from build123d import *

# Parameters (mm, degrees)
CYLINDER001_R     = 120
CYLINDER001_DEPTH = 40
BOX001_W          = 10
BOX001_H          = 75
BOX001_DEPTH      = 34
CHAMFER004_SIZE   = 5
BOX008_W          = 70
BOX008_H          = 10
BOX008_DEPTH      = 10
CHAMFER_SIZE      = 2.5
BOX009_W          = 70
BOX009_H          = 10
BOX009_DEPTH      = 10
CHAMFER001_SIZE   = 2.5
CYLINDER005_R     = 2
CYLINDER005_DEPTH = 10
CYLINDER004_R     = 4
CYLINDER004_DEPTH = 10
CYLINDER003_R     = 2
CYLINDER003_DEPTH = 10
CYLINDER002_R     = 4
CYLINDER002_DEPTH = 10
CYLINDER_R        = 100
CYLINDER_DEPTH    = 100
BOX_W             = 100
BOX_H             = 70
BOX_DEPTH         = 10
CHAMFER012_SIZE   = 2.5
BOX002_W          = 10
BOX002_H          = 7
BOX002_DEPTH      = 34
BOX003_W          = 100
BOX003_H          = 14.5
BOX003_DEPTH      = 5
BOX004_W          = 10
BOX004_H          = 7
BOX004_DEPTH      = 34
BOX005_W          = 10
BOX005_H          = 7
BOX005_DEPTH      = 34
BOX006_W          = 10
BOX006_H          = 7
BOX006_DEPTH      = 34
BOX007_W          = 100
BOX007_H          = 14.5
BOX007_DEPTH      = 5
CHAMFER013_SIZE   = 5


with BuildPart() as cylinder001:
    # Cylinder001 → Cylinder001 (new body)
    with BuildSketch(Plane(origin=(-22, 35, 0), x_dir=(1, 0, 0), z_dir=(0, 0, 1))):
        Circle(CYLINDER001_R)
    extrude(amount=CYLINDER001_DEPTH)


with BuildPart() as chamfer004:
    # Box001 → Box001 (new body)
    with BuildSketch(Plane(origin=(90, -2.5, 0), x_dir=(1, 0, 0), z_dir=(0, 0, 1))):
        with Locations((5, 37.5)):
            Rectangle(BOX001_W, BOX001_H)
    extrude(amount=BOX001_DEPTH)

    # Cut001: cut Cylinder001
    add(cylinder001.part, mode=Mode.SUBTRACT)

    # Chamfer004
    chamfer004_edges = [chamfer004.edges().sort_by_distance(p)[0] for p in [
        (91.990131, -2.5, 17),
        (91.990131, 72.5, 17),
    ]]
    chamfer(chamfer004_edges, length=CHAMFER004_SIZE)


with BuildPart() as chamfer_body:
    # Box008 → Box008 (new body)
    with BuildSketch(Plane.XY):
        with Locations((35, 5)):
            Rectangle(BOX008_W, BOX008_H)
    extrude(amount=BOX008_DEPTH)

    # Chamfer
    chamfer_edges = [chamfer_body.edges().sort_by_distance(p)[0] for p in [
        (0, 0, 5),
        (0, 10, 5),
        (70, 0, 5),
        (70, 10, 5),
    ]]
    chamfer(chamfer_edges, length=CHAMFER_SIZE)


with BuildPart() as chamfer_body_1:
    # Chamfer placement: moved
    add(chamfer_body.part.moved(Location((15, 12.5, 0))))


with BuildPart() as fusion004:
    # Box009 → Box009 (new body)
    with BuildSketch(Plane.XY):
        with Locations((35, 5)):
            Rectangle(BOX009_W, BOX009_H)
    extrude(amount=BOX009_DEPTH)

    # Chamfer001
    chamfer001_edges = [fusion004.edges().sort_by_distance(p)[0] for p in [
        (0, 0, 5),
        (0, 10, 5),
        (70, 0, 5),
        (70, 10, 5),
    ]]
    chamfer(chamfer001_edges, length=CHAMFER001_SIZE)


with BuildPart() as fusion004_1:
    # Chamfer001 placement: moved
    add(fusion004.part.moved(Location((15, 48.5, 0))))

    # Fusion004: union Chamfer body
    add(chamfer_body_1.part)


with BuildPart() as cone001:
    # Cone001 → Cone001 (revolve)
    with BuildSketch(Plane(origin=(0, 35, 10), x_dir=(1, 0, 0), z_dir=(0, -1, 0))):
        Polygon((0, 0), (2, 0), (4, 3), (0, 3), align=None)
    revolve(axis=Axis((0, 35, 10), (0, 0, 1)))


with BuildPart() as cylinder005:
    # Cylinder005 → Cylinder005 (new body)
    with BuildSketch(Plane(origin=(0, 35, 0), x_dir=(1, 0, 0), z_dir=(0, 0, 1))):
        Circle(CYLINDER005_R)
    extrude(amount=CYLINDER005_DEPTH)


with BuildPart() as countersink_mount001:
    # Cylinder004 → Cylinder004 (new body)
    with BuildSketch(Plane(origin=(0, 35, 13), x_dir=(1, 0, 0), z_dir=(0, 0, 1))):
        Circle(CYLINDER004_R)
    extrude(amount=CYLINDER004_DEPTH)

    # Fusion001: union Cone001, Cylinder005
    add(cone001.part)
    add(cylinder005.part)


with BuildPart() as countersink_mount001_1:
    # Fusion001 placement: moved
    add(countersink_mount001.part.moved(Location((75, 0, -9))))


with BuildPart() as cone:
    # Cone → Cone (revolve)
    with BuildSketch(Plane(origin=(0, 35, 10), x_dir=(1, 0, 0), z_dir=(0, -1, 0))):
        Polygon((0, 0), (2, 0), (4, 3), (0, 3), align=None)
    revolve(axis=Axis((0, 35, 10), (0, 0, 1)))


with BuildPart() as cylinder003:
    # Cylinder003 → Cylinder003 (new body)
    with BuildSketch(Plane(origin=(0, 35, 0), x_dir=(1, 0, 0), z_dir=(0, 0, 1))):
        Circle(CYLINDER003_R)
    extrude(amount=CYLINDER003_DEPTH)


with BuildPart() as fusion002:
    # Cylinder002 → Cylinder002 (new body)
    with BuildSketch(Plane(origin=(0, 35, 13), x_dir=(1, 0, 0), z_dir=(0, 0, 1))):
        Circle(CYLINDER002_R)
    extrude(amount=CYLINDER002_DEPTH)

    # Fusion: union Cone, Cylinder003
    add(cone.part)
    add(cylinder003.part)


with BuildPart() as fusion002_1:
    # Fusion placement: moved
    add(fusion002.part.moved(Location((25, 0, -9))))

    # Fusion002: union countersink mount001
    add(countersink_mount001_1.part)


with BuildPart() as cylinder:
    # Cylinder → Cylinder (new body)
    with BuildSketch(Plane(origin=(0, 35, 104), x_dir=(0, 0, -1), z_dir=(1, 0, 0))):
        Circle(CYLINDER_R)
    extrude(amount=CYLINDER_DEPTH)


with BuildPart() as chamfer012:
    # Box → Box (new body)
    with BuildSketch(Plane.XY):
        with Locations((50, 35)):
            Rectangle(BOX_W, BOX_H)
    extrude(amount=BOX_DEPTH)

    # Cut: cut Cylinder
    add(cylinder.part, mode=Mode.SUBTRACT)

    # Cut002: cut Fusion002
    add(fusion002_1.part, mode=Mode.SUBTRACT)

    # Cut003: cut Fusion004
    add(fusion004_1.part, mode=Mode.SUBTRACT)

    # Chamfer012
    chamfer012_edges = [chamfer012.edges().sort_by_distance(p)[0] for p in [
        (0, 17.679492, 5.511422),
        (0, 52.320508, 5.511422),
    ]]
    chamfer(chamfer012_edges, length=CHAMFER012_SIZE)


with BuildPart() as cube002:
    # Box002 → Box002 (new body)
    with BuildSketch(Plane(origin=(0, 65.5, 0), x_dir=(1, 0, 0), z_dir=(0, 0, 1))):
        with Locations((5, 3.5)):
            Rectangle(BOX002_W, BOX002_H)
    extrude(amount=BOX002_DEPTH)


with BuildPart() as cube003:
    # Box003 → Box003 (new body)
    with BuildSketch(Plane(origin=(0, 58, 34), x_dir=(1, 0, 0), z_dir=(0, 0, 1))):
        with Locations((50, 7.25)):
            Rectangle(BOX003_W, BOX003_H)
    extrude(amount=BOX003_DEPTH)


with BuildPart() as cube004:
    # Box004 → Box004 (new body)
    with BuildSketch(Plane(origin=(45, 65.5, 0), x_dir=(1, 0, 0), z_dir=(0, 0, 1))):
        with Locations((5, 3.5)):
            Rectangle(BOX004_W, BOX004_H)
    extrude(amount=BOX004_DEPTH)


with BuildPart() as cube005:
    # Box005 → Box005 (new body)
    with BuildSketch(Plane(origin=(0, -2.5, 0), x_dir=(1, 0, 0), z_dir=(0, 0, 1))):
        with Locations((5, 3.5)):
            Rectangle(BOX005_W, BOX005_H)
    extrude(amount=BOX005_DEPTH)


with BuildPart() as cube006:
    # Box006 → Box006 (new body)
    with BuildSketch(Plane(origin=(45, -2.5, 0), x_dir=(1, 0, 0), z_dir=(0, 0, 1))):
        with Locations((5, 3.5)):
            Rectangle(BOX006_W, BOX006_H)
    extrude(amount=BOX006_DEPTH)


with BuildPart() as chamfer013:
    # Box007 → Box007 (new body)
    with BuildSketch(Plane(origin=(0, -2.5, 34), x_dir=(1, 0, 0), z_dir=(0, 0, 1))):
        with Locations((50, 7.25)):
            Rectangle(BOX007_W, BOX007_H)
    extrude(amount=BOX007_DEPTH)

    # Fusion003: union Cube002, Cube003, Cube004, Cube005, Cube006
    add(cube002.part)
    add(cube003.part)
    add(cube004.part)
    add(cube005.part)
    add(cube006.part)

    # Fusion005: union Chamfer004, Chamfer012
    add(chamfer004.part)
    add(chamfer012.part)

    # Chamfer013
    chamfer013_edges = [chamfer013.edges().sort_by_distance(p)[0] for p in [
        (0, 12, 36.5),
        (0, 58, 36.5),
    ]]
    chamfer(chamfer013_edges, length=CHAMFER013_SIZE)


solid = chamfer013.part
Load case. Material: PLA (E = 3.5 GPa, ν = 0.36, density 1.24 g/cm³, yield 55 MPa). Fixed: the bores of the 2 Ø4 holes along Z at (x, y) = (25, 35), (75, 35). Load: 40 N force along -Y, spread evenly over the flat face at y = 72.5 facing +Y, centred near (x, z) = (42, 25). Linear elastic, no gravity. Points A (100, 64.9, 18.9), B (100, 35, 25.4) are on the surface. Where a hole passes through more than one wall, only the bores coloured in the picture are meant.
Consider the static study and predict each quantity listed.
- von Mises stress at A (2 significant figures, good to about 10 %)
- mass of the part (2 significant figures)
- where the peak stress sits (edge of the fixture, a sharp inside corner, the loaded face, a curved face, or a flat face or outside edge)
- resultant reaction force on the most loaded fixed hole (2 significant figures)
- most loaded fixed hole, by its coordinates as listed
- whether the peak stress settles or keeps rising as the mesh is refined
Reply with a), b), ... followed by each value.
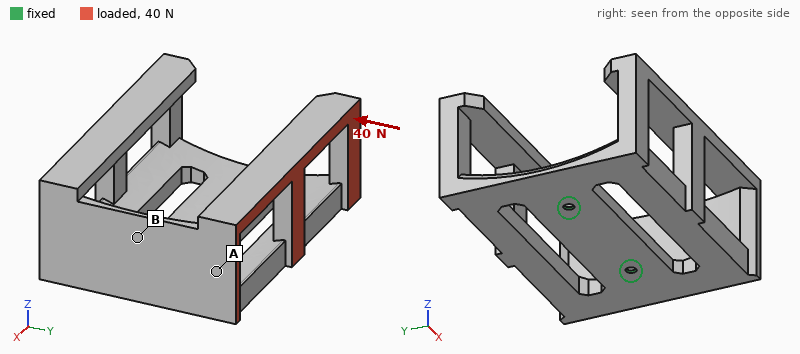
a) 1.5 MPa
b) 80 g
c) edge of the fixture
d) 27 N
e) (25, 35)
f) keeps rising
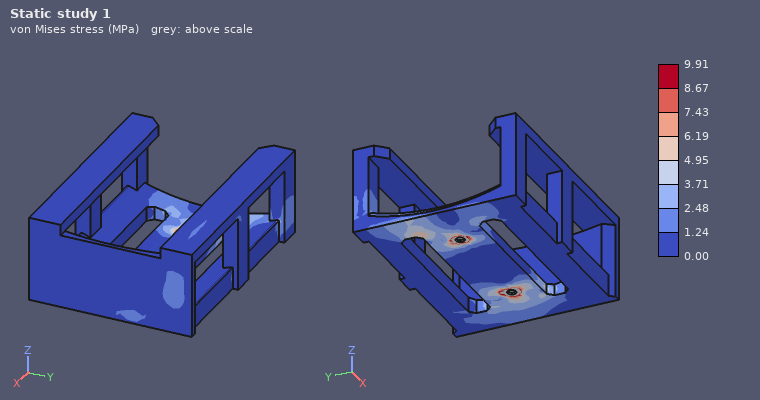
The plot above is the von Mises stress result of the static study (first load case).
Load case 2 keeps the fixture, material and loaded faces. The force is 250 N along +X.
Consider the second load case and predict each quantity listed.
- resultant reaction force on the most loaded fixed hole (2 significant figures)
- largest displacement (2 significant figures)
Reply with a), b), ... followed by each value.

a) 240 N
b) 1.3 mm
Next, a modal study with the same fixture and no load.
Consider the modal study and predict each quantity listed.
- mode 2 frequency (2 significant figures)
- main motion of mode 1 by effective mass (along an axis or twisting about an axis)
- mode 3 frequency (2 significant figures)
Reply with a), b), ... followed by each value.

a) 320 Hz
b) along Y
c) 410 Hz
